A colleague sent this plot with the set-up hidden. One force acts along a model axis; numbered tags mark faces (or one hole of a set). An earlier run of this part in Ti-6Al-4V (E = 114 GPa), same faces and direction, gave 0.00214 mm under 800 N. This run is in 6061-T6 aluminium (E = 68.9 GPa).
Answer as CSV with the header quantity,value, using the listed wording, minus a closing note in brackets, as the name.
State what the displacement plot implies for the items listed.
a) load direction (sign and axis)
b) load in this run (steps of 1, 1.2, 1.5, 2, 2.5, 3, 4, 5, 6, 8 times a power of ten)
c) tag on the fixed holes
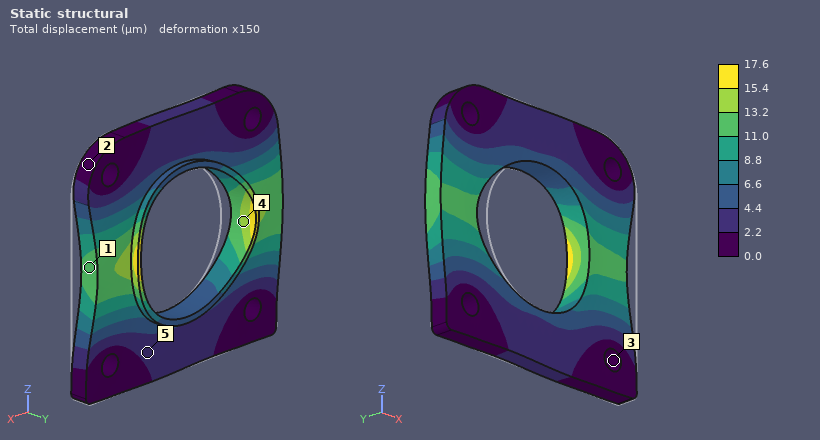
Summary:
quantity,value
load direction,-X
load in this run,4 kN
tag on the fixed holes,3
